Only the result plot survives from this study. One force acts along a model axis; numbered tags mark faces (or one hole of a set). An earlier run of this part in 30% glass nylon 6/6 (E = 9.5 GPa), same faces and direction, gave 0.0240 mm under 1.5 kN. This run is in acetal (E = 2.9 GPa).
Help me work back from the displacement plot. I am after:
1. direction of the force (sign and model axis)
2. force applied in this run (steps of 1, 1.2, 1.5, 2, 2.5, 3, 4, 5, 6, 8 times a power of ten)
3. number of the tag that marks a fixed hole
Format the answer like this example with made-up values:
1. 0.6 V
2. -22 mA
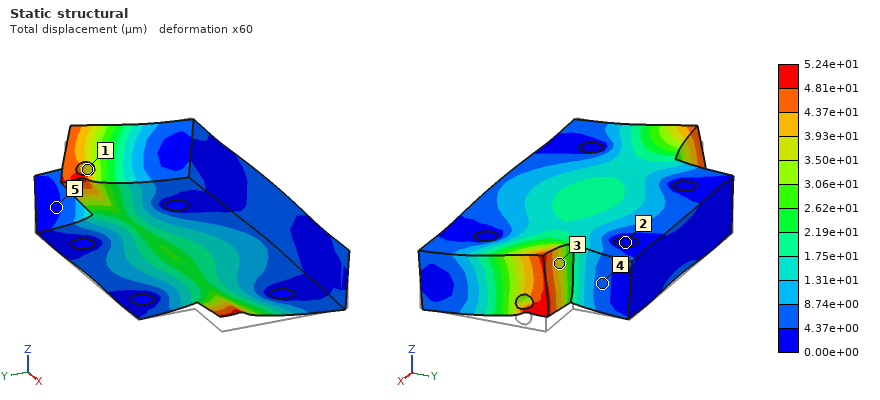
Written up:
1. +Z
2. 1 kN
3. 2
